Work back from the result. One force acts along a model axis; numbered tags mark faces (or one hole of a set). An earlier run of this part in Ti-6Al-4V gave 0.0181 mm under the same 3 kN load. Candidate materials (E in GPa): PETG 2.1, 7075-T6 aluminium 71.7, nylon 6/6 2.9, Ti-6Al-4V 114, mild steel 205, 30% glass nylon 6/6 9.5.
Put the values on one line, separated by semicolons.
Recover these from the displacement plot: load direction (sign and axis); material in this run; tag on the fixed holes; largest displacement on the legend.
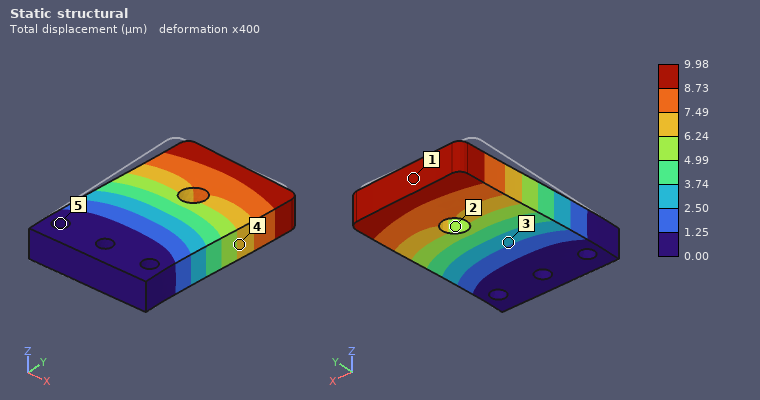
+X; mild steel; 5; 9.98 µm
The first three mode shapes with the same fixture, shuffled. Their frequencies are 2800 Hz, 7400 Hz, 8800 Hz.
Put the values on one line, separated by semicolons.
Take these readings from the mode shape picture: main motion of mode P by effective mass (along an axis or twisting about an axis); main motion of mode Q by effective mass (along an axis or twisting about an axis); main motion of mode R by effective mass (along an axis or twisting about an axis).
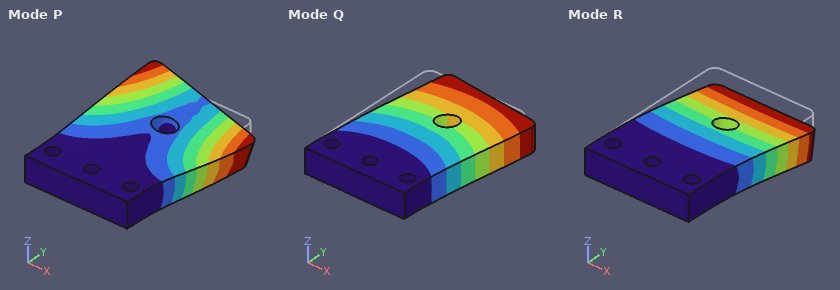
twisting about Y; along X; along Z
